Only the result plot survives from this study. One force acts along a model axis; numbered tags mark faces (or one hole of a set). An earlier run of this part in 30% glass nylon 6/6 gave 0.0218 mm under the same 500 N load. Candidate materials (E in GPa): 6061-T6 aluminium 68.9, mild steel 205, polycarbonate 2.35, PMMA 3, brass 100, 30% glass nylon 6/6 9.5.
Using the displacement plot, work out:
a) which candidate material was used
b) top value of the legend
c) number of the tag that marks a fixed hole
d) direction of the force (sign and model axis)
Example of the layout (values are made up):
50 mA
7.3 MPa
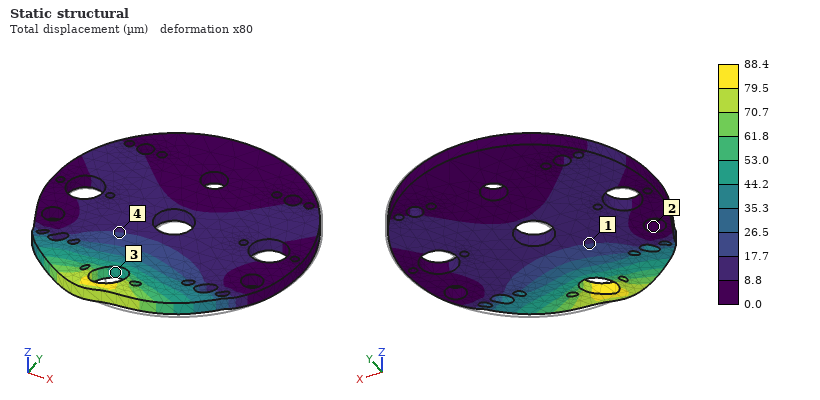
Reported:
polycarbonate
88.4 µm
2
-X
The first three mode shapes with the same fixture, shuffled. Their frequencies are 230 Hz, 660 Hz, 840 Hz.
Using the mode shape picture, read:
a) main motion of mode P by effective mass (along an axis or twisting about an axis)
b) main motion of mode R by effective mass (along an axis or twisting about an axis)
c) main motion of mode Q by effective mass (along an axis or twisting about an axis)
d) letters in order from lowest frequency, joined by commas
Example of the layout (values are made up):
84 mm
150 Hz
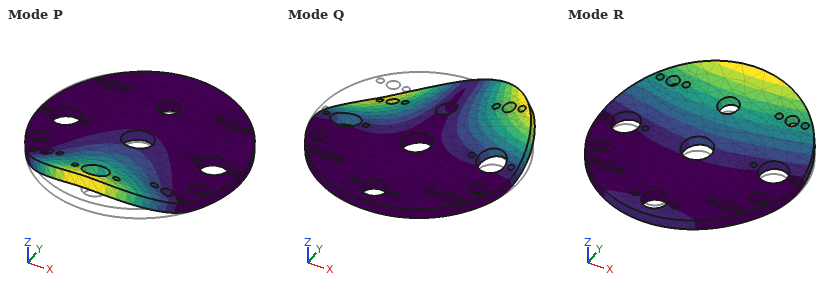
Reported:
along Z
along Z
twisting about Y
R, Q, P
